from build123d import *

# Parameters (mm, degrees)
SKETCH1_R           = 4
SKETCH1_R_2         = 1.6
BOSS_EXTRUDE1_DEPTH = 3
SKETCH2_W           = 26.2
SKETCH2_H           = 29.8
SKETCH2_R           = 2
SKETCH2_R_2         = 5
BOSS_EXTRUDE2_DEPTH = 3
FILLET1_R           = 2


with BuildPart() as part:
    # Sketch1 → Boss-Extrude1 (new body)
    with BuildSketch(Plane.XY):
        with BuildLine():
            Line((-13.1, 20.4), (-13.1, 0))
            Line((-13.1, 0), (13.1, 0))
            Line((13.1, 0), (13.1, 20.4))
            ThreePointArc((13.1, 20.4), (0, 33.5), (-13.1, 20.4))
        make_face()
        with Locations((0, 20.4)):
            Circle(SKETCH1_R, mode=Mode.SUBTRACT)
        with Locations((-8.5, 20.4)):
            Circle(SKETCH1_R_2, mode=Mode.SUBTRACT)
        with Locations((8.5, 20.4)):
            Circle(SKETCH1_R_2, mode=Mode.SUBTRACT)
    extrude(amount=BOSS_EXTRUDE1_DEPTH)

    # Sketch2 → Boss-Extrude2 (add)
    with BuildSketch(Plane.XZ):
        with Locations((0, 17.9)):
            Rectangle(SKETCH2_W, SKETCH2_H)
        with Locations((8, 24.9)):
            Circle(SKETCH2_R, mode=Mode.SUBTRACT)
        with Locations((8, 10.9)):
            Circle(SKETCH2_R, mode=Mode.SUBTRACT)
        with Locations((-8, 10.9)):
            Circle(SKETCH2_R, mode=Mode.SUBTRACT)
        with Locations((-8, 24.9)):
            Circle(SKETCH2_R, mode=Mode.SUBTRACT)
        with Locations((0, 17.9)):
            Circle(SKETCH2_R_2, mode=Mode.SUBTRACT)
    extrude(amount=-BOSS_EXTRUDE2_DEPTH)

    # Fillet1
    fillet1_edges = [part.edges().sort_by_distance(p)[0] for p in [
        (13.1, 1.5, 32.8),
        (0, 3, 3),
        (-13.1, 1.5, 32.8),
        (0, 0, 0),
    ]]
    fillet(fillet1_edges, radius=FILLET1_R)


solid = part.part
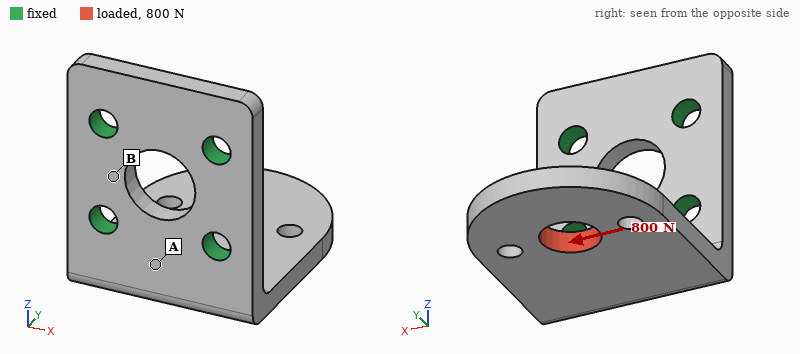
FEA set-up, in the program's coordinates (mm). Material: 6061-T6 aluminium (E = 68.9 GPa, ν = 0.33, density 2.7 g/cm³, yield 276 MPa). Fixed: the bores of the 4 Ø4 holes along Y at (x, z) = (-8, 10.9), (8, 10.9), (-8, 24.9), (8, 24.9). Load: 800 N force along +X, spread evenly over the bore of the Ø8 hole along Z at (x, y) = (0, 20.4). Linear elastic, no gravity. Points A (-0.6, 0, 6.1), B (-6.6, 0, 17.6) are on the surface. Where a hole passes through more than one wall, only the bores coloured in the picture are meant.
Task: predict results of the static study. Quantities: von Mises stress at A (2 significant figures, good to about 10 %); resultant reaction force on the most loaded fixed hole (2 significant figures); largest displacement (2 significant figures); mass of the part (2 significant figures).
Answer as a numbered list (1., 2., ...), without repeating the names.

1. 64 MPa
2. 990 N
3. 0.19 mm
4. 11 g
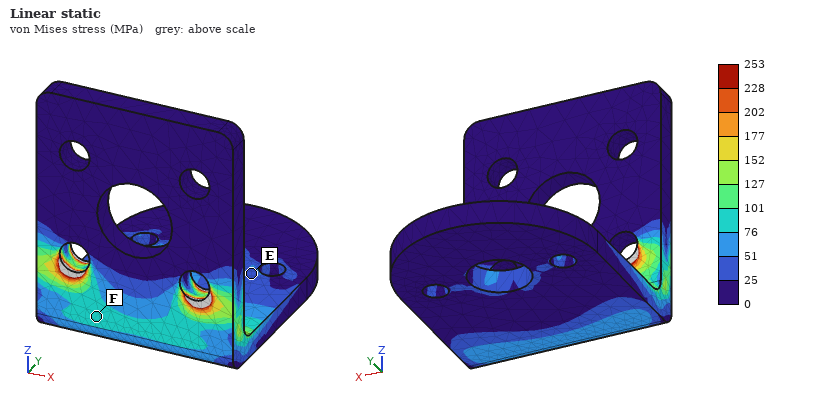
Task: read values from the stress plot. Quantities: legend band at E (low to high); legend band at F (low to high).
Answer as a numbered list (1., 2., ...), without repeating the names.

1. 25 to 51 MPa
2. 76 to 101 MPa
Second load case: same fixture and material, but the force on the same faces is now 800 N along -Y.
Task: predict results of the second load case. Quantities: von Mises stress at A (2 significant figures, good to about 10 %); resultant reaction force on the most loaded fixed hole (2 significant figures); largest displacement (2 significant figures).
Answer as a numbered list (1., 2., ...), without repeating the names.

1. 63 MPa
2. 420 N
3. 0.23 mm
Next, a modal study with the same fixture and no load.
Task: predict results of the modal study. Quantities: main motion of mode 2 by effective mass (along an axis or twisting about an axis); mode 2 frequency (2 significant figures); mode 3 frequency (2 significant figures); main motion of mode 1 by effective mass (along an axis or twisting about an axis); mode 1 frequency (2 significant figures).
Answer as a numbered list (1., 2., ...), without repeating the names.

1. along X
2. 5500 Hz
3. 8300 Hz
4. along Z
5. 2200 Hz
